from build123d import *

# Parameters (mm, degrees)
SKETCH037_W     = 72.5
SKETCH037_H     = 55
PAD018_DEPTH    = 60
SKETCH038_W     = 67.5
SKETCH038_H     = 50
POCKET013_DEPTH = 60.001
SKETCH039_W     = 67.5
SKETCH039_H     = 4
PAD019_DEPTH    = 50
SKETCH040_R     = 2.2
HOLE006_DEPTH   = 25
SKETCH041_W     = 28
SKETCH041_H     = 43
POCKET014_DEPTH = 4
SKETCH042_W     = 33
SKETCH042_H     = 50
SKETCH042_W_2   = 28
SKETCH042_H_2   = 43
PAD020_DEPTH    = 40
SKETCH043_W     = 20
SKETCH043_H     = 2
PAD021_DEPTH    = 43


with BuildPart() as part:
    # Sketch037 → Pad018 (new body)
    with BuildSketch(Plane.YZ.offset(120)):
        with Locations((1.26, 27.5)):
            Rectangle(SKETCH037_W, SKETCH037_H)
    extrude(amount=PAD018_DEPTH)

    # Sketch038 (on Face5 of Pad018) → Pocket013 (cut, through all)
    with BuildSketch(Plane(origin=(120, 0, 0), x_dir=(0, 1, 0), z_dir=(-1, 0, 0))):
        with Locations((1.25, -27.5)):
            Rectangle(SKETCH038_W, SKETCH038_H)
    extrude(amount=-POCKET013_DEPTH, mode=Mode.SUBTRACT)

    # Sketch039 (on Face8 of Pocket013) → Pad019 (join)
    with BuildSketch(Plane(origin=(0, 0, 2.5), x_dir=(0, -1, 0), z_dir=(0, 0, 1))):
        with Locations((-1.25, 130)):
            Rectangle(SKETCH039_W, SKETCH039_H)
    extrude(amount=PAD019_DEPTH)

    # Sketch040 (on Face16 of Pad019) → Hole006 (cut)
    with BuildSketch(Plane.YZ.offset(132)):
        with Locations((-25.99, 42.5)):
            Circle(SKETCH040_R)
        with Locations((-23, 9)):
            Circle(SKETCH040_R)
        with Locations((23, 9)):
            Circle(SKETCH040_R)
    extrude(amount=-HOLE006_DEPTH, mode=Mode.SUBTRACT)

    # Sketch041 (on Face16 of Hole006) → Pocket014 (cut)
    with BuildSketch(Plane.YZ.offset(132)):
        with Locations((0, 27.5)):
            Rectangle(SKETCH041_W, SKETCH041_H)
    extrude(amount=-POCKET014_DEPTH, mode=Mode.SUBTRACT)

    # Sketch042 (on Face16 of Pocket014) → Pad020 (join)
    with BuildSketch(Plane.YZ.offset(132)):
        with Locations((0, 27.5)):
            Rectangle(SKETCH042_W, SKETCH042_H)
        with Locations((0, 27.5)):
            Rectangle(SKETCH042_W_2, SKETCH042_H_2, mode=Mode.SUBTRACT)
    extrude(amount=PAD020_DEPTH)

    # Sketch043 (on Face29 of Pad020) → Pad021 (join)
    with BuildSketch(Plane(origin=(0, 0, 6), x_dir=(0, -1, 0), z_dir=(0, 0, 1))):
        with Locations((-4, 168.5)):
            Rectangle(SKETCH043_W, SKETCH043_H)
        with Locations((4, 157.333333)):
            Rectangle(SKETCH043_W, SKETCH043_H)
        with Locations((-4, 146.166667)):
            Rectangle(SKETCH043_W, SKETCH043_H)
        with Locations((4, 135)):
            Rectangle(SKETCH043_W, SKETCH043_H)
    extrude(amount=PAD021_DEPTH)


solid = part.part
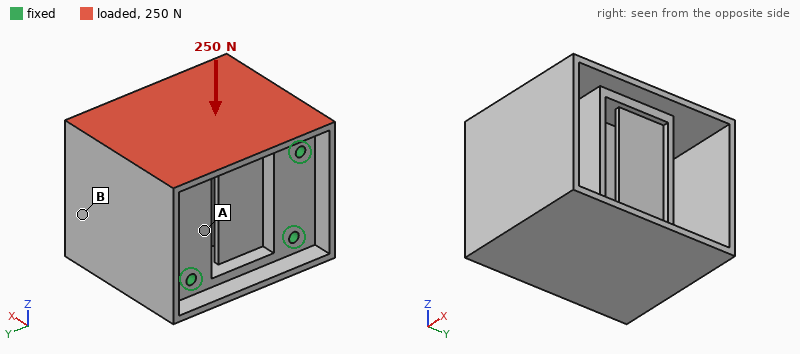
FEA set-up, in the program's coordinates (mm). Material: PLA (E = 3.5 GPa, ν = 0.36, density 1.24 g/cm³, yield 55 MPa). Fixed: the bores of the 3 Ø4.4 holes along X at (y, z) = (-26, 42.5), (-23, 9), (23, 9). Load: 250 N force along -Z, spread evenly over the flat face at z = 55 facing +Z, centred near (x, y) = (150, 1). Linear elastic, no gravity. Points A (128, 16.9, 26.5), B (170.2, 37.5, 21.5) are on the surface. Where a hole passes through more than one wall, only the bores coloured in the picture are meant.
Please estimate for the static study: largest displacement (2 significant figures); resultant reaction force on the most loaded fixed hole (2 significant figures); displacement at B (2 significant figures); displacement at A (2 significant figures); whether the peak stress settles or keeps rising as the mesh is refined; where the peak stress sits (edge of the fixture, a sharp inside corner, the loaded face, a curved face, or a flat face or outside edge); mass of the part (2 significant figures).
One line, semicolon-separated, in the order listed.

0.19 mm; 160 N; 0.11 mm; 0.034 mm; keeps rising; edge of the fixture; 87 g
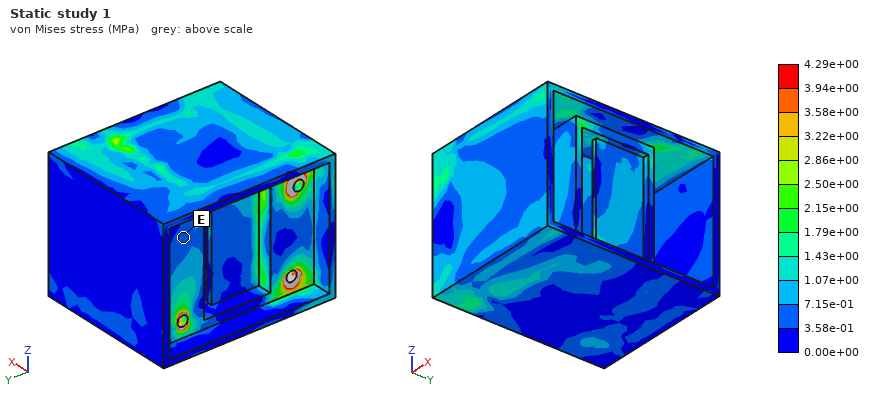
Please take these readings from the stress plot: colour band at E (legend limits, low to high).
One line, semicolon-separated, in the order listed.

3.58e-01 to 7.15e-01 MPa
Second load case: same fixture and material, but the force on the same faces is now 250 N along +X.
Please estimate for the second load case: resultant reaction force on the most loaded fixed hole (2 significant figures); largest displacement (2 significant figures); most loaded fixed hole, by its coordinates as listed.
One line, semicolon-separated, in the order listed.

320 N; 0.40 mm; (-26, 42.5)
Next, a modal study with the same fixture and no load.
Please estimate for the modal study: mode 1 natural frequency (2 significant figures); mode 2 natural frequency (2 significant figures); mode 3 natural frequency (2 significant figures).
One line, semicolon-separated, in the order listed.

710 Hz; 1300 Hz; 1500 Hz
